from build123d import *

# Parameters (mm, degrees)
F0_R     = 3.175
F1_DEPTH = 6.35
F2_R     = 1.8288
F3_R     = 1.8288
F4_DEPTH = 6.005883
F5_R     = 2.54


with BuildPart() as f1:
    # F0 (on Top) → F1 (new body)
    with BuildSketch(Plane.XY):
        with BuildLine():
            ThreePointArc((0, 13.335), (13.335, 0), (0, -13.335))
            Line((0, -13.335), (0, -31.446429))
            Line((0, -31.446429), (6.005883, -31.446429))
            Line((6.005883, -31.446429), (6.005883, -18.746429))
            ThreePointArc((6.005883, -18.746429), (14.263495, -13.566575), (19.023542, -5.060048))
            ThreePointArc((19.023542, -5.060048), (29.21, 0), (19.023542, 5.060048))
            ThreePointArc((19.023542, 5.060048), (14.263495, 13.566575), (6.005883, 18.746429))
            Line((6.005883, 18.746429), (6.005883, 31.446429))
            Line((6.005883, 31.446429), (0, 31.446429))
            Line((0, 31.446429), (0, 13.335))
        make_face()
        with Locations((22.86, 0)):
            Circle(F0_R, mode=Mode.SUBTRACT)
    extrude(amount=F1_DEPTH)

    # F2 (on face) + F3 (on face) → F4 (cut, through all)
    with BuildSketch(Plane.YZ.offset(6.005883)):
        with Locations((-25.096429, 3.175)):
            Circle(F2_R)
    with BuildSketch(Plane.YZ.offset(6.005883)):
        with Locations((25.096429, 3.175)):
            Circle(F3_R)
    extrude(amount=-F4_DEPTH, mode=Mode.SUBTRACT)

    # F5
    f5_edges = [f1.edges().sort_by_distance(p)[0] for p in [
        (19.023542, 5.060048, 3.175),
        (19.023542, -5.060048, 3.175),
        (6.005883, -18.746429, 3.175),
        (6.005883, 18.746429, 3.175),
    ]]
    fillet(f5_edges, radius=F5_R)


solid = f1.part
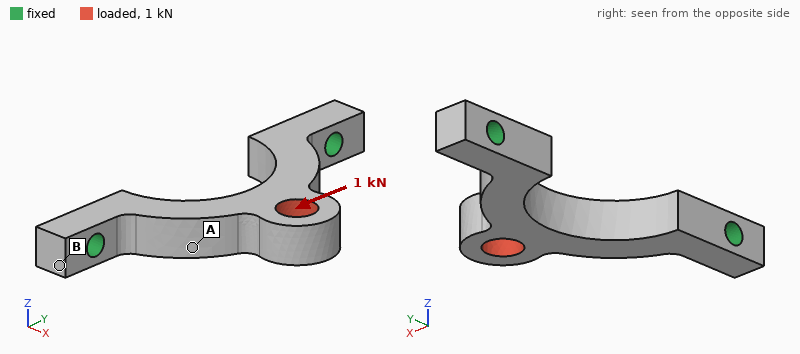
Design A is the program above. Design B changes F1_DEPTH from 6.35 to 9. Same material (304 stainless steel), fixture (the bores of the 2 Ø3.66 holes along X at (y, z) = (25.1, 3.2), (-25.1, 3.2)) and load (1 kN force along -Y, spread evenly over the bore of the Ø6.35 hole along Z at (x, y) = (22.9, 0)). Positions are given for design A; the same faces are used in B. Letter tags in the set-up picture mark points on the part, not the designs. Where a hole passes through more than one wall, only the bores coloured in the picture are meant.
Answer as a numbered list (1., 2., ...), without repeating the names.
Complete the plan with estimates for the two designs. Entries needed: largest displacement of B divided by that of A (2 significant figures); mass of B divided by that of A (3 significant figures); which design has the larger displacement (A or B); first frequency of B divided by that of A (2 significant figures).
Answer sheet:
1. 0.75
2. 1.43
3. A
4. 1.2
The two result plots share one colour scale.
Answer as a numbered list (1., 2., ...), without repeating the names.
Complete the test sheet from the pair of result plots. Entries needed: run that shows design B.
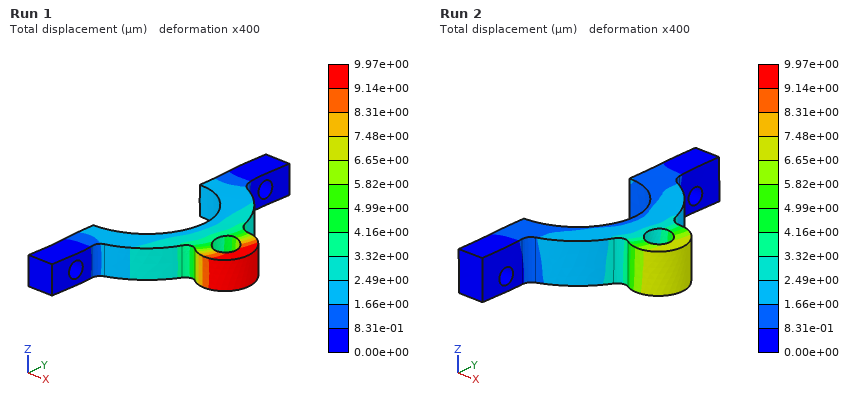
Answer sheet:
1. Run 2
